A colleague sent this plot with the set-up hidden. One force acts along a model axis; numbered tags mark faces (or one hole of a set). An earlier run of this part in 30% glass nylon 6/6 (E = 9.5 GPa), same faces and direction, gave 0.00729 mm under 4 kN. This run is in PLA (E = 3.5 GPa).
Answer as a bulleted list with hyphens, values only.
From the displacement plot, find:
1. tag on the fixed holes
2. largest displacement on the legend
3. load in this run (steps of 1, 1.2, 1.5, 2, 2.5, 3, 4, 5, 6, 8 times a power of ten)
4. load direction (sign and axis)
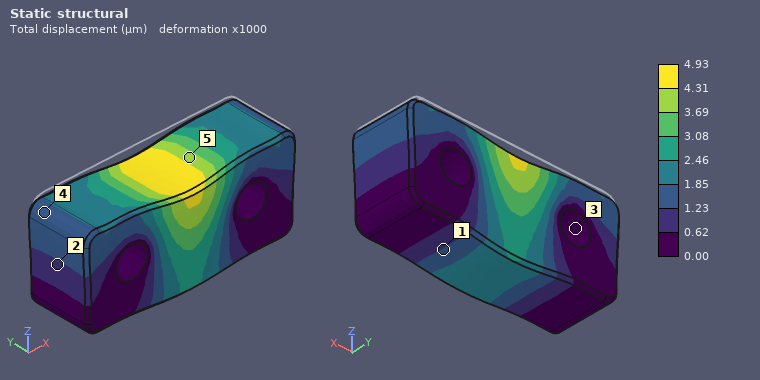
- 3
- 4.93 µm
- 1 kN
- -Z
